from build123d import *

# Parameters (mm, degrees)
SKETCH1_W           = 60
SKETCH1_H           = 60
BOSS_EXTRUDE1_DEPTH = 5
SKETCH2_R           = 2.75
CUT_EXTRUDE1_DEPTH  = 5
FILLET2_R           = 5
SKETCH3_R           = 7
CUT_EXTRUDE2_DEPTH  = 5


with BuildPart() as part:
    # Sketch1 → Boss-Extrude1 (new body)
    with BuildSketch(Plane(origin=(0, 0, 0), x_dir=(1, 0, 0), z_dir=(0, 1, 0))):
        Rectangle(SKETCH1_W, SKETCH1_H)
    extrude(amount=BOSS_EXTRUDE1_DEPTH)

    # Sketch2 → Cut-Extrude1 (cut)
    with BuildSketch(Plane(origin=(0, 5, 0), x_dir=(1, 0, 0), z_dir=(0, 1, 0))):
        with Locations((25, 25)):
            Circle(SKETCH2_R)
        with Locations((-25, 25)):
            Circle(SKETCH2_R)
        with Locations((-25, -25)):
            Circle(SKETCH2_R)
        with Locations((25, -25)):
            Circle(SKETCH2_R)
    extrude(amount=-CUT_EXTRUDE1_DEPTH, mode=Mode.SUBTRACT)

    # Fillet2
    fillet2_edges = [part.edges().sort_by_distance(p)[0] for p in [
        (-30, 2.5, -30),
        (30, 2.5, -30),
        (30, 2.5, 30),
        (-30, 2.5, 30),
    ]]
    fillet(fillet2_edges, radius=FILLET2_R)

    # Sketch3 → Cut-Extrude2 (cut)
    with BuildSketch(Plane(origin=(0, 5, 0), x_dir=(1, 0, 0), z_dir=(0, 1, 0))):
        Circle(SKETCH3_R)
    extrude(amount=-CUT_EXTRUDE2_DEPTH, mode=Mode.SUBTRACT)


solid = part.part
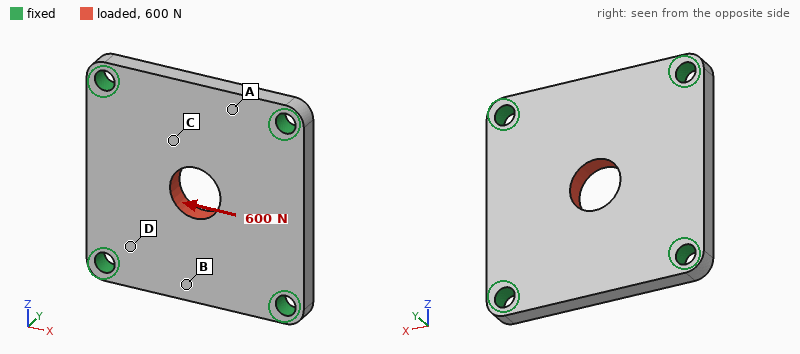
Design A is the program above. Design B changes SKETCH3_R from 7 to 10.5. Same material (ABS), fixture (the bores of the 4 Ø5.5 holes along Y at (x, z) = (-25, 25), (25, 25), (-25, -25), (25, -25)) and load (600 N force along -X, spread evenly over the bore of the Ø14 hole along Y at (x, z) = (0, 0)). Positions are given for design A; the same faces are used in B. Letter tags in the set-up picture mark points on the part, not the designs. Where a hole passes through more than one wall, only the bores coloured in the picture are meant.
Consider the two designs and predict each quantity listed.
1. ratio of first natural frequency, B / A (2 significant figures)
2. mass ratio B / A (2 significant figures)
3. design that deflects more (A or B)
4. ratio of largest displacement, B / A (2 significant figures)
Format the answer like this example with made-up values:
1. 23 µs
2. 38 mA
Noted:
1. 1.1
2. 0.94
3. A
4. 0.92
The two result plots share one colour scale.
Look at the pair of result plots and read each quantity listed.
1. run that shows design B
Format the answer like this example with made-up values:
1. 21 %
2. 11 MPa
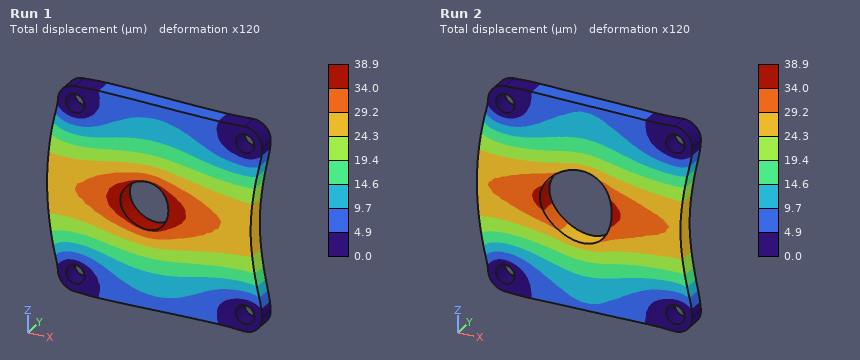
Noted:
1. Run 2
